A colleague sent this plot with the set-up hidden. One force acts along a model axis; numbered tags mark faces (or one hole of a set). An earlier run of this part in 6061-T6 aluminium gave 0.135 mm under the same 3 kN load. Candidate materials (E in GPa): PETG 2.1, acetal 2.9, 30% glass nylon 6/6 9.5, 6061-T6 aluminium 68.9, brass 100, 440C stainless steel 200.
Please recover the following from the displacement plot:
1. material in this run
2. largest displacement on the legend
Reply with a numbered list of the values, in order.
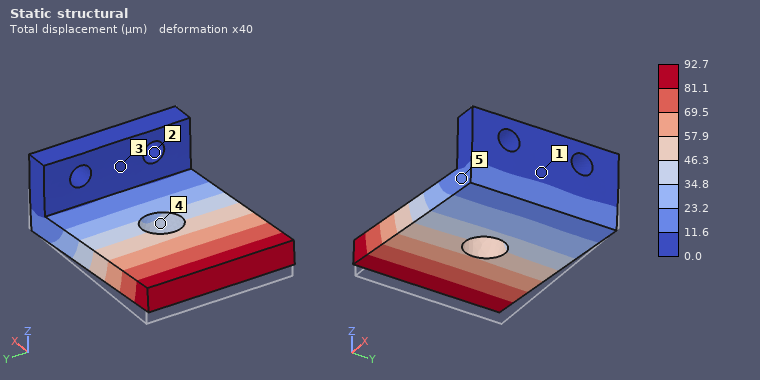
1. brass
2. 92.7 µm
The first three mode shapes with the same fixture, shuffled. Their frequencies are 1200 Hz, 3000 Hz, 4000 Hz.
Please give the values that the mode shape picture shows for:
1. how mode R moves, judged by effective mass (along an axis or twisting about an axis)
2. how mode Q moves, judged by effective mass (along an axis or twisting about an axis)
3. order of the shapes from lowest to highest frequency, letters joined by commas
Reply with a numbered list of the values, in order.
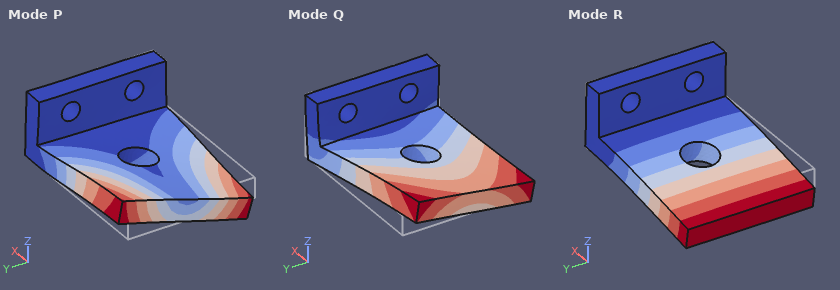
1. along Z
2. along Y
3. R, Q, P
